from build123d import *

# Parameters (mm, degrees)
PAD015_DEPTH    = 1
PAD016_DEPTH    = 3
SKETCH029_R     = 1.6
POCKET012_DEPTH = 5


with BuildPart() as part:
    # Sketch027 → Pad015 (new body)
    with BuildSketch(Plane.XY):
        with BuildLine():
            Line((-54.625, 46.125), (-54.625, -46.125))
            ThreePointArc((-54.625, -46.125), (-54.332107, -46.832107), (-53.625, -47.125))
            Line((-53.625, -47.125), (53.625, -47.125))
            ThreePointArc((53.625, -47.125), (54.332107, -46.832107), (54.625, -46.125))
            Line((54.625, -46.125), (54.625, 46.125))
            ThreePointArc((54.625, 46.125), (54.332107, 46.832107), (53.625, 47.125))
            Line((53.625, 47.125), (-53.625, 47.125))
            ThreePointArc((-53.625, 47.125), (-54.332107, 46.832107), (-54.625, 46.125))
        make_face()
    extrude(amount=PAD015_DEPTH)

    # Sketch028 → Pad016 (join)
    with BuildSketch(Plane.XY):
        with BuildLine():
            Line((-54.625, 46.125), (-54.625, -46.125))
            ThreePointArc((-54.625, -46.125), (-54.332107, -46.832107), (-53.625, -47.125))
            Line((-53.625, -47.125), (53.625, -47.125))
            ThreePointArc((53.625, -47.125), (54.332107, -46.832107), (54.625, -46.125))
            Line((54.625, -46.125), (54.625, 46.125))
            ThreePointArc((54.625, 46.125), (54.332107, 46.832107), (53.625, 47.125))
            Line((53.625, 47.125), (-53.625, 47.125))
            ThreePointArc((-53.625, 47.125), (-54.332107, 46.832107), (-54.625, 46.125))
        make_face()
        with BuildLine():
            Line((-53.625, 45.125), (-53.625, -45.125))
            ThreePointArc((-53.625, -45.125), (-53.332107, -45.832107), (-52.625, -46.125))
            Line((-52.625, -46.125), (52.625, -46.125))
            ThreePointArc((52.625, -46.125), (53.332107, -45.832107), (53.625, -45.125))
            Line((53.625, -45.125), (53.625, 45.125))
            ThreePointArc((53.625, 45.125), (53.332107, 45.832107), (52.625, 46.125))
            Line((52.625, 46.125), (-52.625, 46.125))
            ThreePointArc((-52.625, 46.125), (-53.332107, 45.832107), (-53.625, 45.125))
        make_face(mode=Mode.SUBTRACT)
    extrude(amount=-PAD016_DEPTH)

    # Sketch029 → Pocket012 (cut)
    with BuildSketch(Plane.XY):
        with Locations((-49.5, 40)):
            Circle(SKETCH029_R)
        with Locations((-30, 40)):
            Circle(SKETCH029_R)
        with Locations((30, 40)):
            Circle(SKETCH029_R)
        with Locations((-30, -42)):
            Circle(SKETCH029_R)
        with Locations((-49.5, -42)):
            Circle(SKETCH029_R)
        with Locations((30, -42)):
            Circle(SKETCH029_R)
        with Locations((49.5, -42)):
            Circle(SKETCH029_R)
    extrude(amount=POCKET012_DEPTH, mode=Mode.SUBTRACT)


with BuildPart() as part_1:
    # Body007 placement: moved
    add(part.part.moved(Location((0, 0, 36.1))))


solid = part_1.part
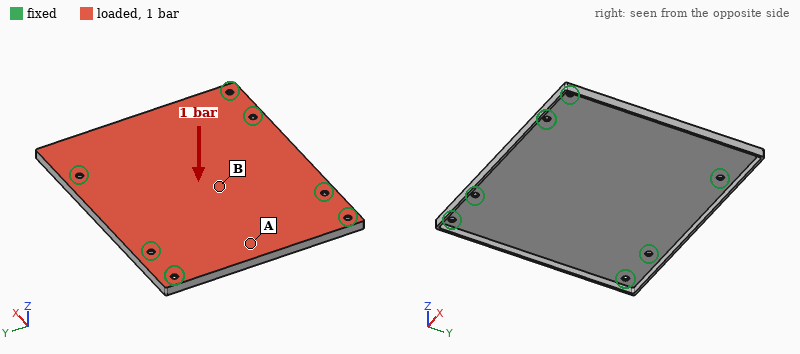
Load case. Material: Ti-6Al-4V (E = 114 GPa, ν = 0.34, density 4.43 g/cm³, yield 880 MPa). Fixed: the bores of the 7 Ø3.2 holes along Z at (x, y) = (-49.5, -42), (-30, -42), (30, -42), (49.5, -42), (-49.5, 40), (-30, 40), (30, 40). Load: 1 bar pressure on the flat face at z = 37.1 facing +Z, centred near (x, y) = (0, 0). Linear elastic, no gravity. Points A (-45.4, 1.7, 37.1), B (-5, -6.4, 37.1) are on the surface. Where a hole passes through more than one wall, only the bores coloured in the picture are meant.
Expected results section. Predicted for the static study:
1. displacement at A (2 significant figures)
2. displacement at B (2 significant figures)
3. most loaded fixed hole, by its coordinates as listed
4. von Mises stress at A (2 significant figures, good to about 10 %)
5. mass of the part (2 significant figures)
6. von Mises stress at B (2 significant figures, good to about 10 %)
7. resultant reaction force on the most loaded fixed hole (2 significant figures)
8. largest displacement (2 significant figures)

0.58 mm
1.6 mm
(30, 40)
79 MPa
51 g
160 MPa
280 N
1.6 mm
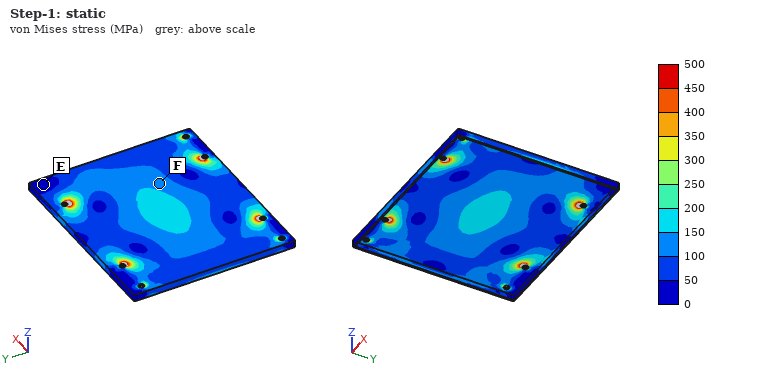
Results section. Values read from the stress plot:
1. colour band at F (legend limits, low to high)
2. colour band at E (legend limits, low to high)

100 to 150 MPa
0 to 50 MPa
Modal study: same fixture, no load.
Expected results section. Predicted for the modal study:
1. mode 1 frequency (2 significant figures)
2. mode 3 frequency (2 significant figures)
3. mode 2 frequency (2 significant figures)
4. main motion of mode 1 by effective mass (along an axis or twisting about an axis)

740 Hz
1400 Hz
1100 Hz
along Z
